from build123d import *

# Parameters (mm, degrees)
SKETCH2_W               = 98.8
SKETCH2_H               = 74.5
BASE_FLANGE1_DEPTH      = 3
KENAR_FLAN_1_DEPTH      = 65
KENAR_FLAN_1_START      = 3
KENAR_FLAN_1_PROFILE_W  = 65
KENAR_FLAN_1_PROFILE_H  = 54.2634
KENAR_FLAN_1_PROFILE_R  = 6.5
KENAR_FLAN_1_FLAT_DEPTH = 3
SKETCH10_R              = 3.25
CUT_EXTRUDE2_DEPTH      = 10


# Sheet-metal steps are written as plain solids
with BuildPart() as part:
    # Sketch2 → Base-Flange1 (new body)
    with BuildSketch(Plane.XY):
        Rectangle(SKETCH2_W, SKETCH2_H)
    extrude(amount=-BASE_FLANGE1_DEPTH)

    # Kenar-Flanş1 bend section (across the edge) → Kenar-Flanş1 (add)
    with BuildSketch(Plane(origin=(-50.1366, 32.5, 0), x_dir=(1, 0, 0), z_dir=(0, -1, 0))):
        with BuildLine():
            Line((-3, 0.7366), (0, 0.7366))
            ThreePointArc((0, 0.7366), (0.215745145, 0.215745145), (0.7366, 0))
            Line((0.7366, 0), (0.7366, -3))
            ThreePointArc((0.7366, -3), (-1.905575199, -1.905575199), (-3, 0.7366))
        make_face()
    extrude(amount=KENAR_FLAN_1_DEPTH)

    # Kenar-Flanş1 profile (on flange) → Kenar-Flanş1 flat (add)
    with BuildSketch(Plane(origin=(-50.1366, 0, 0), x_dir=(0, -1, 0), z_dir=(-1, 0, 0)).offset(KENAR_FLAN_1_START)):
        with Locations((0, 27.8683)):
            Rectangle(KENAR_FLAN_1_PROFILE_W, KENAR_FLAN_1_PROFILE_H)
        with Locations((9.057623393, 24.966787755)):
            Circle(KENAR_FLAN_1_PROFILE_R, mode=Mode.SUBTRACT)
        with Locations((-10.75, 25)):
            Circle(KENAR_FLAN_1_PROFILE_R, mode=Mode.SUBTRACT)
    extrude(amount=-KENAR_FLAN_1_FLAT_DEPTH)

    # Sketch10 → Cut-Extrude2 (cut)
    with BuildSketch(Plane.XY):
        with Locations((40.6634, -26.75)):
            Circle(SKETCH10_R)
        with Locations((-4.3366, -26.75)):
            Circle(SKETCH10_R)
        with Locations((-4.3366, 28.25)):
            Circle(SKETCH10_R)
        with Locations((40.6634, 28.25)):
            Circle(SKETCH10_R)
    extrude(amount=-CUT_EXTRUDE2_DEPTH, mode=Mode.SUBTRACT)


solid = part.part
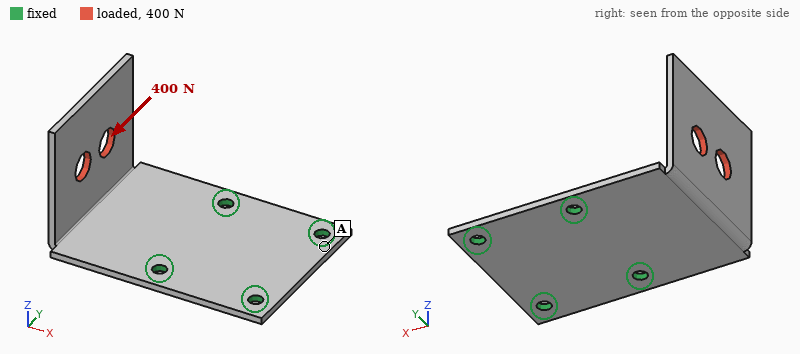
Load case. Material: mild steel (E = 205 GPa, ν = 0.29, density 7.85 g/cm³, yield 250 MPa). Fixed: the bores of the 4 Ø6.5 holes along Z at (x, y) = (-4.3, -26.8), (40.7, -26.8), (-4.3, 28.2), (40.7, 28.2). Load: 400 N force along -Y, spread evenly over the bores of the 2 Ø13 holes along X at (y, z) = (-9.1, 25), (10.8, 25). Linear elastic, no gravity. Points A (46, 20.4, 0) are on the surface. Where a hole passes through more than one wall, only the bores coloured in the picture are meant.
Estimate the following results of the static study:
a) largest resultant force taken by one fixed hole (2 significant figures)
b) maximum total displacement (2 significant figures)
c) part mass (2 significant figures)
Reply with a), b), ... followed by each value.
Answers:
a) 410 N
b) 0.32 mm
c) 250 g
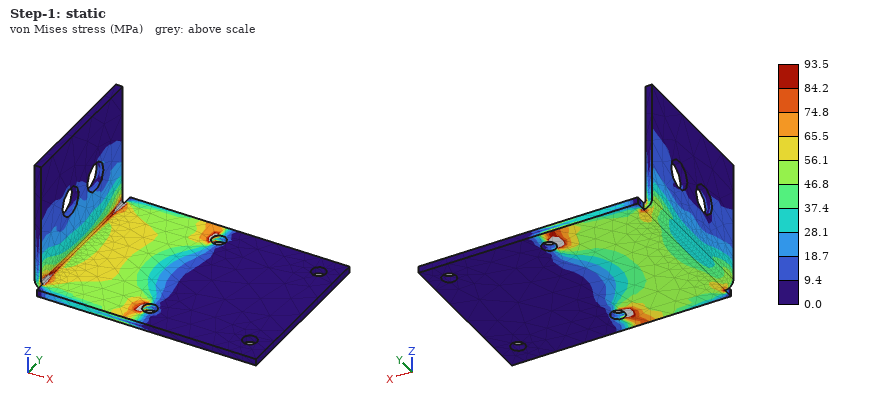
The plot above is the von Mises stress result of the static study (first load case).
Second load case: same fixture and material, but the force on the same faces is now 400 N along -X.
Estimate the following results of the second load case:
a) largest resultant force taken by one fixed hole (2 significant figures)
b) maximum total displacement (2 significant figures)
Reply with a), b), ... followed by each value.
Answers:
a) 170 N
b) 1.1 mm
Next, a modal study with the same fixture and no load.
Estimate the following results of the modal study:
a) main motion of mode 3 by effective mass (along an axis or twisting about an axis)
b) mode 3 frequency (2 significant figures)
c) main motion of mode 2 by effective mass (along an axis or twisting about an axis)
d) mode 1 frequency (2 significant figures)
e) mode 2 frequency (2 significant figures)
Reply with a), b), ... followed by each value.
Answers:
a) along Z
b) 870 Hz
c) along Y
d) 340 Hz
e) 660 Hz
